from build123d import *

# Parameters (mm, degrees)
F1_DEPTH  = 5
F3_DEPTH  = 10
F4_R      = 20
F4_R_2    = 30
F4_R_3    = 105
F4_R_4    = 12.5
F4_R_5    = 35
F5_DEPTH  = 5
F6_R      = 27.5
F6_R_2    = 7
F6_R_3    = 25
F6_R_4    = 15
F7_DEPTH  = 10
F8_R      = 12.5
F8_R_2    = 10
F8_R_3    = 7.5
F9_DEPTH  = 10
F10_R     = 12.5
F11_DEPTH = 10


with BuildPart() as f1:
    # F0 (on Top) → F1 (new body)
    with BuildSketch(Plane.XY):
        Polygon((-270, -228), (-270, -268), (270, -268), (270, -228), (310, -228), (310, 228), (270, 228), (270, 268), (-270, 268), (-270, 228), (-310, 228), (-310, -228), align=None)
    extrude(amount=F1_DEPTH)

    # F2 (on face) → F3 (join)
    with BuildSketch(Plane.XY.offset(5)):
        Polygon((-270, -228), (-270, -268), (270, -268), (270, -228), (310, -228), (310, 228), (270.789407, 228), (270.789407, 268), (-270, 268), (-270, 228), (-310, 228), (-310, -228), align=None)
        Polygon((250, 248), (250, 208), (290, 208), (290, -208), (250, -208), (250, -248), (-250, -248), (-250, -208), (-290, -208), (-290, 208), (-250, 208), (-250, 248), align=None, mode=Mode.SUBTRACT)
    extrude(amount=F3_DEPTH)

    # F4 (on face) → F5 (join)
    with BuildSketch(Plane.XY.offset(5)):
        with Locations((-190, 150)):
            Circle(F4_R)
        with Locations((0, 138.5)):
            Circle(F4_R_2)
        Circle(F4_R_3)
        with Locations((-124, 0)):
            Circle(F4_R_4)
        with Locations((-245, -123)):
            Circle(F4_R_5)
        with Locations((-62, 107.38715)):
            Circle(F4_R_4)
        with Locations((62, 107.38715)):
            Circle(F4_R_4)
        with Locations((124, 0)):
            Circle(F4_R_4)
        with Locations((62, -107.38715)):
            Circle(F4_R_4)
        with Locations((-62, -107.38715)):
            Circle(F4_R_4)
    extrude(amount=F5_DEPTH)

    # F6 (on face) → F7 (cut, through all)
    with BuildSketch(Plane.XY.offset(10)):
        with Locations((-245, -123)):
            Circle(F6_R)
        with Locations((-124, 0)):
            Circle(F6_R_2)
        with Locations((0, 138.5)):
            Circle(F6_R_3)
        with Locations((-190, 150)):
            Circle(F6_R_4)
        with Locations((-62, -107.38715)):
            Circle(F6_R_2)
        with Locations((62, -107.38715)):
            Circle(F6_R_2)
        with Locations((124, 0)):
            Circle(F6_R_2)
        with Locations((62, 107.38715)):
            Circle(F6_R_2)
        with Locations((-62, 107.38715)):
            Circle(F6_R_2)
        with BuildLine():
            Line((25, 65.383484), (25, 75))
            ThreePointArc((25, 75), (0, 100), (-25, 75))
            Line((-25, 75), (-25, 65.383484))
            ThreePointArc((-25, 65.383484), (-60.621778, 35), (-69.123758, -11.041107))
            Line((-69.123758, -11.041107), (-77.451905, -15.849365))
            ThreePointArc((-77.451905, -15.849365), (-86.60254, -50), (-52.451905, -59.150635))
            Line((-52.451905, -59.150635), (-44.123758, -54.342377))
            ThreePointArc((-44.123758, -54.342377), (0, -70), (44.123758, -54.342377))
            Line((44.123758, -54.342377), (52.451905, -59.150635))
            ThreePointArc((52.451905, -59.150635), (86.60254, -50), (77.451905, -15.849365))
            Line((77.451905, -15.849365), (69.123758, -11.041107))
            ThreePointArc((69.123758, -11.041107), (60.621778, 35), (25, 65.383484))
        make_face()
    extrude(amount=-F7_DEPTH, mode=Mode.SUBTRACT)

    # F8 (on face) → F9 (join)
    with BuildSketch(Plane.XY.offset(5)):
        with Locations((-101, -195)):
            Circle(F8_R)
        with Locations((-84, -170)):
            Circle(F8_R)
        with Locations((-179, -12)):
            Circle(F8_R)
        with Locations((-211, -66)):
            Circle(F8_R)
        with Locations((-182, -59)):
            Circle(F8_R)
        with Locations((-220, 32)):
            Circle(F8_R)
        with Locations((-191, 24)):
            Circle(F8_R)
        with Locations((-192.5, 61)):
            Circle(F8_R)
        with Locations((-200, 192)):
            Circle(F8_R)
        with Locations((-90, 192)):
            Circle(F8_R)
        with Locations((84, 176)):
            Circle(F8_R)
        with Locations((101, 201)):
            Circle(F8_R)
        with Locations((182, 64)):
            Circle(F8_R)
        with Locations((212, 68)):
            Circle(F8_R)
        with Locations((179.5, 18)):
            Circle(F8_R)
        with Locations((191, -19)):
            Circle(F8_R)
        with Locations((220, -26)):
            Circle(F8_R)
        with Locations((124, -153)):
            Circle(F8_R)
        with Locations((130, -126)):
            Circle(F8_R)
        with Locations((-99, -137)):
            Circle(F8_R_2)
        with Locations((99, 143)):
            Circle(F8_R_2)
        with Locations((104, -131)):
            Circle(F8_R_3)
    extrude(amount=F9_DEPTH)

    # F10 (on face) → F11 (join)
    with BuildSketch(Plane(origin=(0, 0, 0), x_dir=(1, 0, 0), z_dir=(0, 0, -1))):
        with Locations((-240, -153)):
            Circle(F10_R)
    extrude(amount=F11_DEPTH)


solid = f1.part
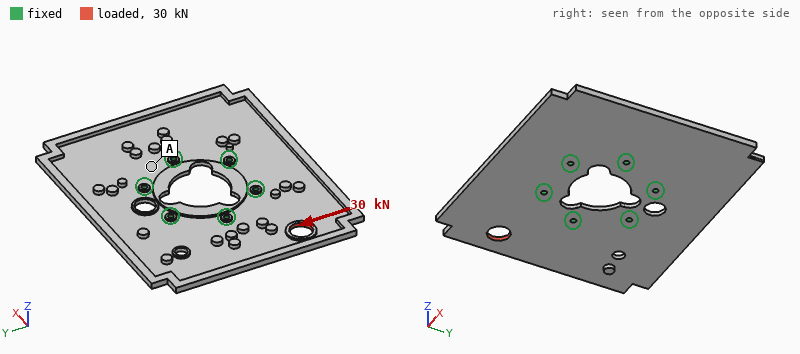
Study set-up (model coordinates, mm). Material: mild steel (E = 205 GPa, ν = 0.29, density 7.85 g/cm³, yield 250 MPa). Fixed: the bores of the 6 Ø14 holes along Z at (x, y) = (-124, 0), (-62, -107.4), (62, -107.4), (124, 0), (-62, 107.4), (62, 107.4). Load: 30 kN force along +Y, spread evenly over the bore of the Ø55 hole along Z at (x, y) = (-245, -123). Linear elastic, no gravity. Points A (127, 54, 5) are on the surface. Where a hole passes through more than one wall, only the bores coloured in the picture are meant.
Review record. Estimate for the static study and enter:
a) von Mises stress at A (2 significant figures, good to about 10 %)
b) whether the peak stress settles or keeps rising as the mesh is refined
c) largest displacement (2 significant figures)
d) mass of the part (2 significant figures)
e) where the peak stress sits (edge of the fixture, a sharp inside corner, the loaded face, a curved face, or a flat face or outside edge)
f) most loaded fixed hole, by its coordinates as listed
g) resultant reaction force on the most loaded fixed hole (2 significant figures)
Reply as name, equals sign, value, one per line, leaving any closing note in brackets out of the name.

von Mises stress at A = 7.1 MPa
whether the peak stress settles or keeps rising as the mesh is refined = keeps rising
largest displacement = 0.68 mm
mass of the part = 17 kg
where the peak stress sits = edge of the fixture
most loaded fixed hole, by its coordinates as listed = (-124, 0)
resultant reaction force on the most loaded fixed hole = 20 kN
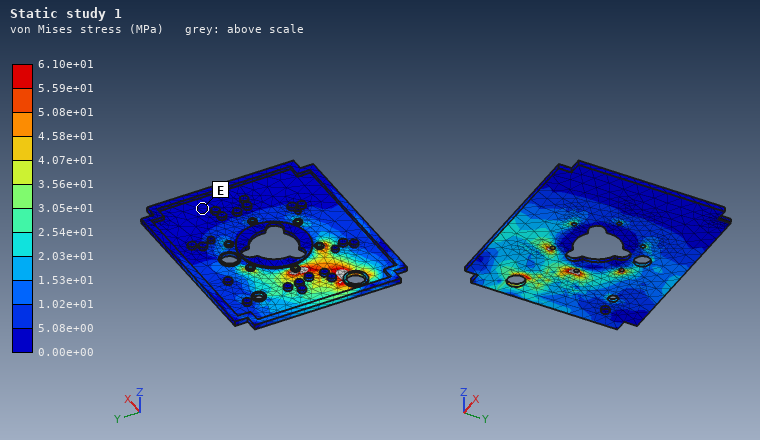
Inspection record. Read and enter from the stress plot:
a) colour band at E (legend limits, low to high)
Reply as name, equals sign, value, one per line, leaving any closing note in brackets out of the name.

colour band at E = 0.00e+00 to 5.08e+00 MPa
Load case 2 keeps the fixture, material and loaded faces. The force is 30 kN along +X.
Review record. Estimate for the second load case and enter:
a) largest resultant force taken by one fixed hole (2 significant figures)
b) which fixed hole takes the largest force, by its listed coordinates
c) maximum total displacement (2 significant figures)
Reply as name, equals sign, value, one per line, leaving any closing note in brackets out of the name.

largest resultant force taken by one fixed hole = 16 kN
which fixed hole takes the largest force, by its listed coordinates = (-62, -107.4)
maximum total displacement = 0.81 mm
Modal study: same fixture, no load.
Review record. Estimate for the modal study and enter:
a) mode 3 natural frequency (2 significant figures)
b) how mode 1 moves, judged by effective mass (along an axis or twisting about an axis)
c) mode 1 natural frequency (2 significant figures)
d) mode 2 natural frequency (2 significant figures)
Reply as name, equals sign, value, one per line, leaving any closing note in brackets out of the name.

mode 3 natural frequency = 92 Hz
how mode 1 moves, judged by effective mass = twisting about Y
mode 1 natural frequency = 76 Hz
mode 2 natural frequency = 89 Hz
